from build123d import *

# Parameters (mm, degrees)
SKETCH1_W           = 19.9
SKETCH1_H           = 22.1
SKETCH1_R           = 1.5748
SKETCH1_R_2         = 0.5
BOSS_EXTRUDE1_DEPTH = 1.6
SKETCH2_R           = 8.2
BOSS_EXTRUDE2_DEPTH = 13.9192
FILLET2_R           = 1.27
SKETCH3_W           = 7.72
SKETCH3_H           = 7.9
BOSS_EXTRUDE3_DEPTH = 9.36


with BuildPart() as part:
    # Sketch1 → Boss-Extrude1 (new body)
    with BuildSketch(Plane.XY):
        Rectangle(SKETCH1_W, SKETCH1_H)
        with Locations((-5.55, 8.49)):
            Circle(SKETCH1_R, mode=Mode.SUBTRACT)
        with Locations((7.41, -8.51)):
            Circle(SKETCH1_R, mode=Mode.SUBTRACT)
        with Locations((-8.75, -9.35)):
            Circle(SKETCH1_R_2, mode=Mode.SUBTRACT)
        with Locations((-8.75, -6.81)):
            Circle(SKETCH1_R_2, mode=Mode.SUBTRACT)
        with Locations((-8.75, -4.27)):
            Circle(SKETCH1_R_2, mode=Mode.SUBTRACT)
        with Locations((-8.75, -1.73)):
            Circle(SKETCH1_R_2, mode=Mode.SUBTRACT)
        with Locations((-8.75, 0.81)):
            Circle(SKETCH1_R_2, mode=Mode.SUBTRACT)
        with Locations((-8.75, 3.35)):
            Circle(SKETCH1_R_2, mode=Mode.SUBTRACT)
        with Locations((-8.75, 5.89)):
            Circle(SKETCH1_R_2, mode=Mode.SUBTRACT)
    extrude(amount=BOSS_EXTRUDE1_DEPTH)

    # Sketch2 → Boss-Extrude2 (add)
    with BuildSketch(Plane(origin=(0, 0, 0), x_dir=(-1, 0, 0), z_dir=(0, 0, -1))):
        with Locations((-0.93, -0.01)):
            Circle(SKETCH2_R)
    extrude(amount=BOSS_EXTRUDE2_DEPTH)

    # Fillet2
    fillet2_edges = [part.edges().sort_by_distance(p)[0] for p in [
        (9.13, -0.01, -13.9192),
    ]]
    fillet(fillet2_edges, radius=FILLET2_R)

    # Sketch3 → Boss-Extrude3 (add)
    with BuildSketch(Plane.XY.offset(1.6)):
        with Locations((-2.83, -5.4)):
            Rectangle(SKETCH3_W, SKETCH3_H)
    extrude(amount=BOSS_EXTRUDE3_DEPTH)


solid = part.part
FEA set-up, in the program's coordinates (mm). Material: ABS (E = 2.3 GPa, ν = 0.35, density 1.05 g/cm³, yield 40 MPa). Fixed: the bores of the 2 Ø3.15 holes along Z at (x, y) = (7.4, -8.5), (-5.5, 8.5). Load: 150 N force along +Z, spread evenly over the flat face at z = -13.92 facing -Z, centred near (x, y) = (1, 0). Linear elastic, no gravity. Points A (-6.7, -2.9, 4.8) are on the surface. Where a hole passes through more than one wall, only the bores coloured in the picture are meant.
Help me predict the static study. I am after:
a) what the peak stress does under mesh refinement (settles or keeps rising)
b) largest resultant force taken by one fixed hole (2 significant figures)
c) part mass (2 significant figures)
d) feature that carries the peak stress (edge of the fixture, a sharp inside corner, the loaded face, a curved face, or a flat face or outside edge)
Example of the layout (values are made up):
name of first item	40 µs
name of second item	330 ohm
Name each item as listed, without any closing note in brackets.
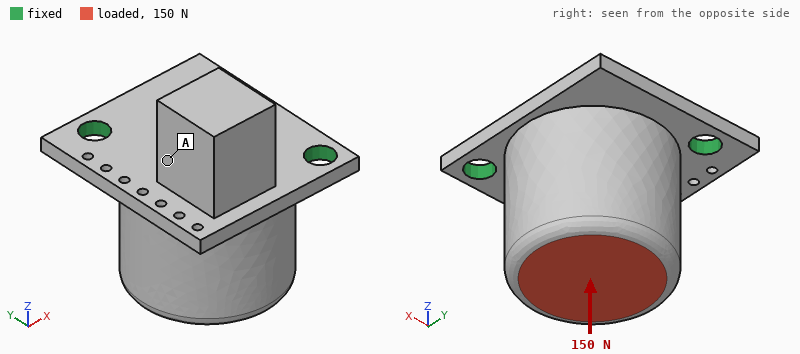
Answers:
what the peak stress does under mesh refinement	keeps rising
largest resultant force taken by one fixed hole	84 N
part mass	4.4 g
feature that carries the peak stress	edge of the fixture
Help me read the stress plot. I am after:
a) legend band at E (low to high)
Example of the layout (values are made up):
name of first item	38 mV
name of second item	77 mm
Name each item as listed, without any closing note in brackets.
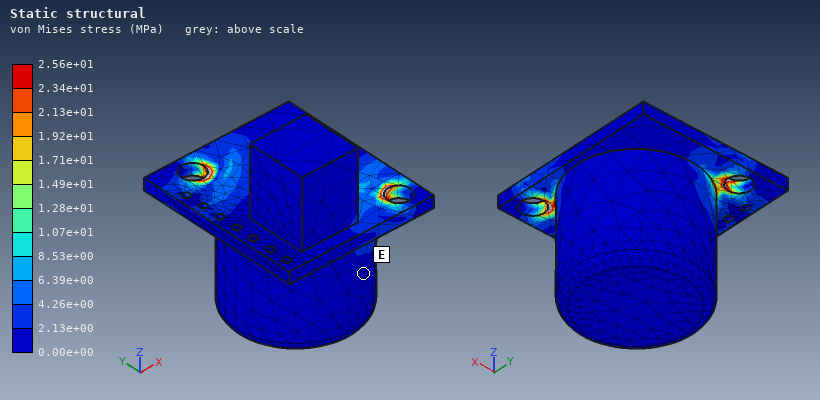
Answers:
legend band at E	0.00e+00 to 2.13e+00 MPa
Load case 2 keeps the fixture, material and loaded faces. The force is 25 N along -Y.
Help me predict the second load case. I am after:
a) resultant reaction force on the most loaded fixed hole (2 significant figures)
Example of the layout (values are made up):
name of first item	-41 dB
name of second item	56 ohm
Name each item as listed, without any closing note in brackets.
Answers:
resultant reaction force on the most loaded fixed hole	21 N
